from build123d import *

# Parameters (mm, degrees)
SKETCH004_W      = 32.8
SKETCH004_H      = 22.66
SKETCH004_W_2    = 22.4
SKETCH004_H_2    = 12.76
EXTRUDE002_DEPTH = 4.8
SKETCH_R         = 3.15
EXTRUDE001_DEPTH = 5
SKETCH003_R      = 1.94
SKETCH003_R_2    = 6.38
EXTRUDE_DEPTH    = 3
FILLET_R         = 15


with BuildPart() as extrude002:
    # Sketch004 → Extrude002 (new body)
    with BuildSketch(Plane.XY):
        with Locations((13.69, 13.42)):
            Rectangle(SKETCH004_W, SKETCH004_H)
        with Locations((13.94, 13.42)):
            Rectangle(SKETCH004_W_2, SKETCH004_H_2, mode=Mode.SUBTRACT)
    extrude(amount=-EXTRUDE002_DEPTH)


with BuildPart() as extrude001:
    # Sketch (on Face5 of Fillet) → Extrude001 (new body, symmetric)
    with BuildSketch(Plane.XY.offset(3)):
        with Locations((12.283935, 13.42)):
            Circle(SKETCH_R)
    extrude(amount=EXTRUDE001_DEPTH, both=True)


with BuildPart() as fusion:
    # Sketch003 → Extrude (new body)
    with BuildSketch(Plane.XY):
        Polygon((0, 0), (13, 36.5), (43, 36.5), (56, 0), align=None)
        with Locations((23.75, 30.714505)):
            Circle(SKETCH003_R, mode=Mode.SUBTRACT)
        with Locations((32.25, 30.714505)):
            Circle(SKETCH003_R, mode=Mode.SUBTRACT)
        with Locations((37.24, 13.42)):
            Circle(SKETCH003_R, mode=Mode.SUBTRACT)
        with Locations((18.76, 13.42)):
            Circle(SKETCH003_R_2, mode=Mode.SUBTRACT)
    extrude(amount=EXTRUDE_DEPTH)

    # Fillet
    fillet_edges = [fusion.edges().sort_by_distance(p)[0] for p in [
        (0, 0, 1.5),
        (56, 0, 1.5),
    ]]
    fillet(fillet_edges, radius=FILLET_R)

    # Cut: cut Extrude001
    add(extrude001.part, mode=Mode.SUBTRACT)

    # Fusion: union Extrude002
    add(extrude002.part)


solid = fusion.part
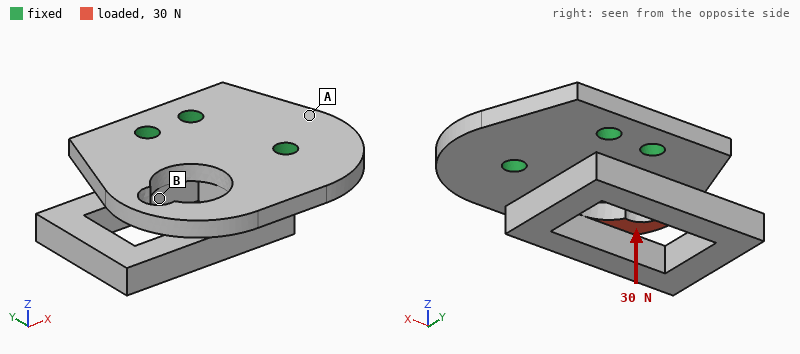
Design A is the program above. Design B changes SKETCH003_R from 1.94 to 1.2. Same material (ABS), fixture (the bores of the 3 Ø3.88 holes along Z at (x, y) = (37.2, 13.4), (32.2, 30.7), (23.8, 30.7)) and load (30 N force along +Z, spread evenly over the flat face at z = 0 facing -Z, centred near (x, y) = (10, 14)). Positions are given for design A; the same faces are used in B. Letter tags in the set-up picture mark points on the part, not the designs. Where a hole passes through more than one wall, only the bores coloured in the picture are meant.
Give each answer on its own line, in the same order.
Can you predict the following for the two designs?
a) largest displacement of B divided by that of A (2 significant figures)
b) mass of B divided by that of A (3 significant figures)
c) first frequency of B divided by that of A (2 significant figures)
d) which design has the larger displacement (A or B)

1.2
1.01
0.91
B
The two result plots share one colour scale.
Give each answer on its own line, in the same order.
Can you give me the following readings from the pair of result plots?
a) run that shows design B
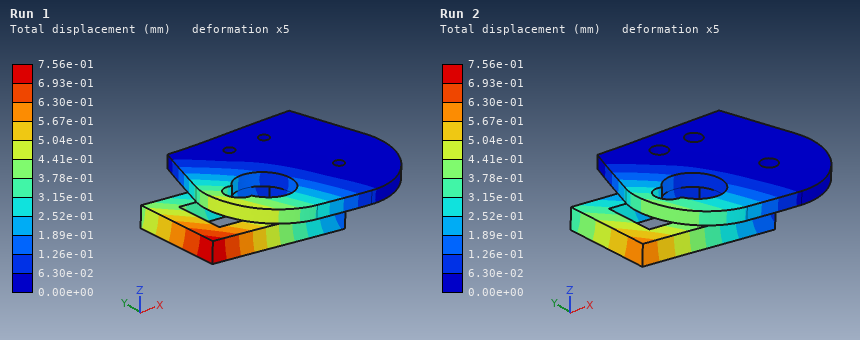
Run 1
